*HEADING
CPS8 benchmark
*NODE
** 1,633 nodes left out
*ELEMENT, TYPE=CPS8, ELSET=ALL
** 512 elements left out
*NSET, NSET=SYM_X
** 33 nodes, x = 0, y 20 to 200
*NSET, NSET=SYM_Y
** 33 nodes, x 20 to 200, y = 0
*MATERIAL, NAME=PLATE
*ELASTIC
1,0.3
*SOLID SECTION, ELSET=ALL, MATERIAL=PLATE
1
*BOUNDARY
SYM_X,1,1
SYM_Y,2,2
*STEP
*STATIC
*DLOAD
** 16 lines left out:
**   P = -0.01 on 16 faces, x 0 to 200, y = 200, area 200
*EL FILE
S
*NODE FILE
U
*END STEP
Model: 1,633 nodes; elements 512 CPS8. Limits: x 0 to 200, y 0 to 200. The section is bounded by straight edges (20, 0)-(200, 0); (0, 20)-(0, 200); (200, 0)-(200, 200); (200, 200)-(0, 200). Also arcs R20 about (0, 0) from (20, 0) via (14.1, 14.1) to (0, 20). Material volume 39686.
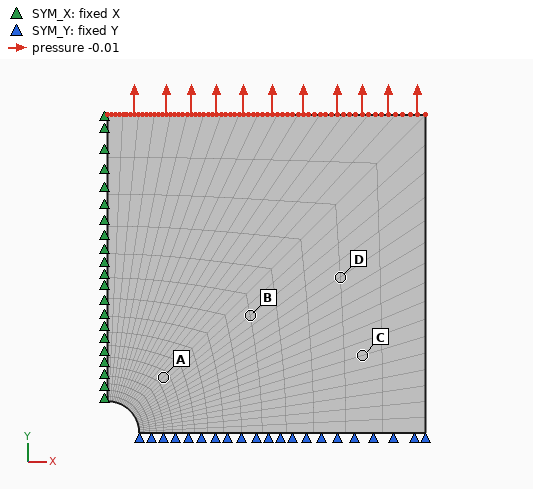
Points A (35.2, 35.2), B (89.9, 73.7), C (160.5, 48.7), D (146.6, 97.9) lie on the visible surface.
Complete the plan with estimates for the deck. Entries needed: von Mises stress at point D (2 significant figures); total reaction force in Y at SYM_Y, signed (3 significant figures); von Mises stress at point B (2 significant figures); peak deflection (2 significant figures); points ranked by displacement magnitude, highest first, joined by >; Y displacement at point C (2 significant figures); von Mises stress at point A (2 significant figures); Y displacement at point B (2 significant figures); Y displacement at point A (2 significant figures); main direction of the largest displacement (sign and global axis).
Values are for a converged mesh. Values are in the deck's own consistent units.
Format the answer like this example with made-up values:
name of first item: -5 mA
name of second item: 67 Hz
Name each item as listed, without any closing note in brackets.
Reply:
von Mises stress at point D: 0.010
total reaction force in Y at SYM_Y, signed: -2.00
von Mises stress at point B: 0.011
peak deflection: 2.1
points ranked by displacement magnitude, highest first, joined by >: D > B > C > A
Y displacement at point C: 0.49
von Mises stress at point A: 0.012
Y displacement at point B: 0.77
Y displacement at point A: 0.45
main direction of the largest displacement: +Y
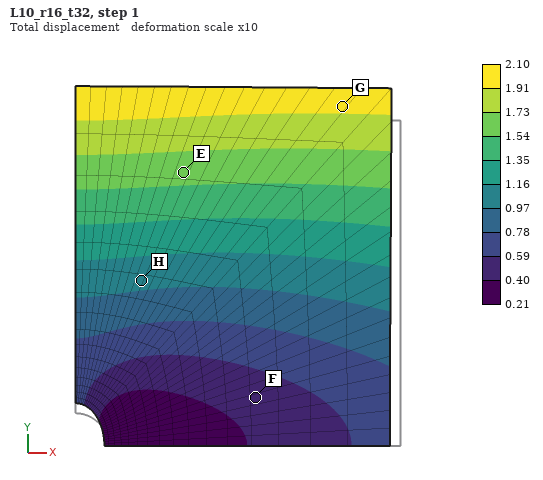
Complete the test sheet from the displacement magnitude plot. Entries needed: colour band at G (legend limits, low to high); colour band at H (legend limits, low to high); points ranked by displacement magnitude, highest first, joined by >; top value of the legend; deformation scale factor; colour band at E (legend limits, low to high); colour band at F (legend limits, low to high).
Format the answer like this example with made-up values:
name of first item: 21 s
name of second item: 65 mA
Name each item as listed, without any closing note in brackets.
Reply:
colour band at G: 1.91 to 2.10
colour band at H: 0.97 to 1.16
points ranked by displacement magnitude, highest first, joined by >: G > E > H > F
top value of the legend: 2.10
deformation scale factor: 10
colour band at E: 1.54 to 1.73
colour band at F: 0.40 to 0.59
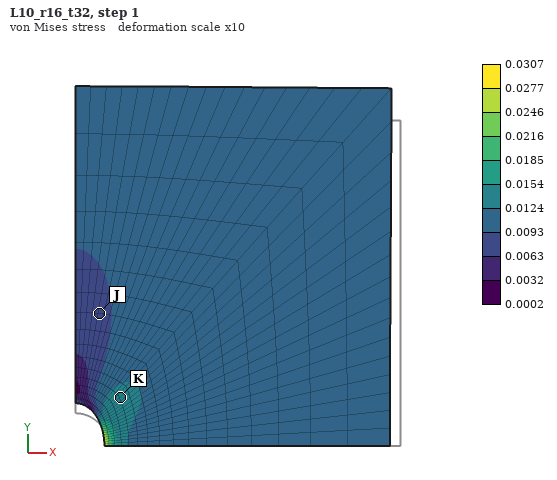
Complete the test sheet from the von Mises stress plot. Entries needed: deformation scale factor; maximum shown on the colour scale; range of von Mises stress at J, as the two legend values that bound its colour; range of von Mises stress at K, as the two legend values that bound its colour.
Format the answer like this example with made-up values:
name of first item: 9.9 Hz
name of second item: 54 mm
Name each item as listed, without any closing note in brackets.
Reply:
deformation scale factor: 10
maximum shown on the colour scale: 0.0307
range of von Mises stress at J, as the two legend values that bound its colour: 0.0063 to 0.0093
range of von Mises stress at K, as the two legend values that bound its colour: 0.0124 to 0.0154
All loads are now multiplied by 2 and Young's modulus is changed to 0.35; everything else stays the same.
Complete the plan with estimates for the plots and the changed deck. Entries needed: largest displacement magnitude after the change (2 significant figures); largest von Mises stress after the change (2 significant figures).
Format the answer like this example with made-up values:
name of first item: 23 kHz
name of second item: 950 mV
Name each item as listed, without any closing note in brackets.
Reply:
largest displacement magnitude after the change: 12
largest von Mises stress after the change: 0.061
